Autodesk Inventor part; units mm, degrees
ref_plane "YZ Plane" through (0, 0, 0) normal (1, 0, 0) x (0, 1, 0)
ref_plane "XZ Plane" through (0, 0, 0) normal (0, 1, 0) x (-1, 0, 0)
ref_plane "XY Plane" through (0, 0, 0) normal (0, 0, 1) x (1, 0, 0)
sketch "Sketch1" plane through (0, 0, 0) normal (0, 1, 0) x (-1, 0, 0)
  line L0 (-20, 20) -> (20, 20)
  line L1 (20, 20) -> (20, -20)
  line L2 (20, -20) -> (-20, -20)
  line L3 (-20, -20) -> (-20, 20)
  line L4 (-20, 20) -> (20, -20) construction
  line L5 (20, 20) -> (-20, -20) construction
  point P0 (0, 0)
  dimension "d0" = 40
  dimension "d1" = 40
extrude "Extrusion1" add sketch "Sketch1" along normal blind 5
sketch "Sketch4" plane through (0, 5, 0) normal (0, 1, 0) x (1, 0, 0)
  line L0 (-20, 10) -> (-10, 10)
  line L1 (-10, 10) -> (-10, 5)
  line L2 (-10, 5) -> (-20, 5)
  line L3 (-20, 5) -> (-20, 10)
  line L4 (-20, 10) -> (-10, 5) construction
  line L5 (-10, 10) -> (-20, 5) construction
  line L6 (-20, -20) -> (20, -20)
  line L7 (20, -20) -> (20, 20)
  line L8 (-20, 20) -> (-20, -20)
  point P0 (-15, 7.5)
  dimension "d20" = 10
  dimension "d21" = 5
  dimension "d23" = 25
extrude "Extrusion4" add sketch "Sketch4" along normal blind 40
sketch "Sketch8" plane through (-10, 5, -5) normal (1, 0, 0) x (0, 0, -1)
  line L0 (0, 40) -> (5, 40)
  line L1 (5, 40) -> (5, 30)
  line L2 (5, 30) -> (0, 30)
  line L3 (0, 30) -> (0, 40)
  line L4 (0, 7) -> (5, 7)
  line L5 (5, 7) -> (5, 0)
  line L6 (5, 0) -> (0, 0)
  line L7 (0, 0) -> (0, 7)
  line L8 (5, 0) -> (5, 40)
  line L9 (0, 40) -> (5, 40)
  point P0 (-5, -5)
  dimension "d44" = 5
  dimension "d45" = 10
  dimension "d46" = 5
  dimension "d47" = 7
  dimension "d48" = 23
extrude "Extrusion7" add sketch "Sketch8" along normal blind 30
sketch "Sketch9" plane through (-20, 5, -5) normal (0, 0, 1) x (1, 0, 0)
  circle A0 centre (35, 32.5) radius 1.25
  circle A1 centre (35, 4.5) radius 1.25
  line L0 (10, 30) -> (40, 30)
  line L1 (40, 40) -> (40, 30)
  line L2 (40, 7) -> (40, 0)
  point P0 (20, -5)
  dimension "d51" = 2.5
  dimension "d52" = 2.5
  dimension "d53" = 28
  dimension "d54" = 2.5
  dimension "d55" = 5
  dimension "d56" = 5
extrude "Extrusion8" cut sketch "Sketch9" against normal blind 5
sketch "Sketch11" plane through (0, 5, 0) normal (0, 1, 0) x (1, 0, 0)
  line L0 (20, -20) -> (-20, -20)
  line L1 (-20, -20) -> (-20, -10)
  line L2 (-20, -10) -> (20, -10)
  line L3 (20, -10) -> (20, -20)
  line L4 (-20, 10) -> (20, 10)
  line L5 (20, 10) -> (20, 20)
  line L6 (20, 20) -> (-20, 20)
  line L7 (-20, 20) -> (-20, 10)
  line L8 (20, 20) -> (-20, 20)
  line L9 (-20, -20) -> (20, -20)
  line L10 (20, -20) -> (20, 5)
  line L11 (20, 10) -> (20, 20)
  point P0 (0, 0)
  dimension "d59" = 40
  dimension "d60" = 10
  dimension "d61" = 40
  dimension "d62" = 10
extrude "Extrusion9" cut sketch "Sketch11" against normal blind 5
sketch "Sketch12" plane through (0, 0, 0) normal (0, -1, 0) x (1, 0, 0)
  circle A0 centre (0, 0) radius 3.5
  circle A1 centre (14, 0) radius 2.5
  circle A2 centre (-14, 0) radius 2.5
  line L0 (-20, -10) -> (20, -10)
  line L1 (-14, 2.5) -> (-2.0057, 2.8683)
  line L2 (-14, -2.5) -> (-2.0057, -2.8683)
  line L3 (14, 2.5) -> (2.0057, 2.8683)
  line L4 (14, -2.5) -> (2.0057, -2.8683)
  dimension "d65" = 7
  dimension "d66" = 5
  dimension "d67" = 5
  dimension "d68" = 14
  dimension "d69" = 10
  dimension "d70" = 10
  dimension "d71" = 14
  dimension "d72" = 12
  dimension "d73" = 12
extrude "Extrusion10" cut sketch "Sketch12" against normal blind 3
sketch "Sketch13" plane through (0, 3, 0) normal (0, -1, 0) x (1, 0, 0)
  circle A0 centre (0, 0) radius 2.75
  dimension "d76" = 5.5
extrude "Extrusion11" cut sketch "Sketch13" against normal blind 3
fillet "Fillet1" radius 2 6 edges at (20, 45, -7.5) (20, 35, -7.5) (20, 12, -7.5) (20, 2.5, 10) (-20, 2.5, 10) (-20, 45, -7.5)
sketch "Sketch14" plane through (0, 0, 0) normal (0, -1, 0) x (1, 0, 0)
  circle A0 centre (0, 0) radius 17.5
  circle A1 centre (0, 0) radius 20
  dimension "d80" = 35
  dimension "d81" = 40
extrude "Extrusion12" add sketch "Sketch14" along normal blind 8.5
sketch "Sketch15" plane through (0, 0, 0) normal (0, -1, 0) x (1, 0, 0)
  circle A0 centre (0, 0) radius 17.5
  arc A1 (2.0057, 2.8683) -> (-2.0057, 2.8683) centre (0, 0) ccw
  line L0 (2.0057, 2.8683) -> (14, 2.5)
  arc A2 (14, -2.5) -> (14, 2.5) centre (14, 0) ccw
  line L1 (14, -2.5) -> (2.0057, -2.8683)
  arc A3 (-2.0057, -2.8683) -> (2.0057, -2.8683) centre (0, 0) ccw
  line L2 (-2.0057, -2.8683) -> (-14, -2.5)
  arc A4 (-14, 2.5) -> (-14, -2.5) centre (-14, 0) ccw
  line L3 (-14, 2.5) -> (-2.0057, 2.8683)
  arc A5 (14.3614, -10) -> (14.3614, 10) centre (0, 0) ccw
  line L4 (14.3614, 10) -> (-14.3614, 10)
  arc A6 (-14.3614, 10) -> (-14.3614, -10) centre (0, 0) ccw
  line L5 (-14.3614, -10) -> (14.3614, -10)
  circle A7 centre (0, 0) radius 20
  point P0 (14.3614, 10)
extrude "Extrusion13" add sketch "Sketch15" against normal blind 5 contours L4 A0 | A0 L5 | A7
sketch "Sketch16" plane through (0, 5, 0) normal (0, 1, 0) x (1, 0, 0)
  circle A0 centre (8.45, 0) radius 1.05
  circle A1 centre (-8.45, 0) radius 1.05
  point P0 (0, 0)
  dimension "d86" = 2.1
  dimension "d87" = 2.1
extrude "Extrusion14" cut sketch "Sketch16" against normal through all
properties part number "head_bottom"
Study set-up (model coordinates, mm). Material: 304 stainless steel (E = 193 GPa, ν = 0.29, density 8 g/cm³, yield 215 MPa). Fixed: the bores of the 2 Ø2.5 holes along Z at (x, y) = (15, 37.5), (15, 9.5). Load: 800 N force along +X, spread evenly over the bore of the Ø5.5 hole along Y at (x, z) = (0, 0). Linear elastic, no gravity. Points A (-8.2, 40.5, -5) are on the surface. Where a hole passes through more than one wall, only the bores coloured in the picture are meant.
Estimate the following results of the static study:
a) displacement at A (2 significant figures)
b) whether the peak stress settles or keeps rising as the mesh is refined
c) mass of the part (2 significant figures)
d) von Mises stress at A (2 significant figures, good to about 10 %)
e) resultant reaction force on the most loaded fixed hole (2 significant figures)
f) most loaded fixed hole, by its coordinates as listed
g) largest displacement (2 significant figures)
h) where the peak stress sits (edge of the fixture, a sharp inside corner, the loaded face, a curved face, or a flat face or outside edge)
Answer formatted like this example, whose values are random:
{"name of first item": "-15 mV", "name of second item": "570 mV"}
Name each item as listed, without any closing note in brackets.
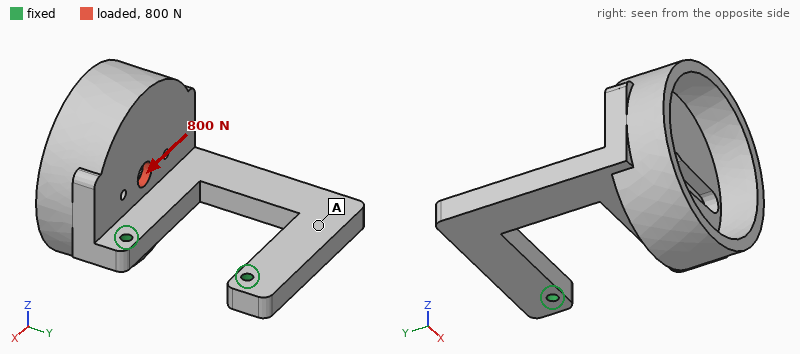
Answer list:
{"displacement at A": "9.7 µm", "whether the peak stress settles or keeps rising as the mesh is refined": "keeps rising", "mass of the part": "100 g", "von Mises stress at A": "10.0 MPa", "resultant reaction force on the most loaded fixed hole": "860 N", "most loaded fixed hole, by its coordinates as listed": "(15, 9.5)", "largest displacement": "44 µm", "where the peak stress sits": "edge of the fixture"}
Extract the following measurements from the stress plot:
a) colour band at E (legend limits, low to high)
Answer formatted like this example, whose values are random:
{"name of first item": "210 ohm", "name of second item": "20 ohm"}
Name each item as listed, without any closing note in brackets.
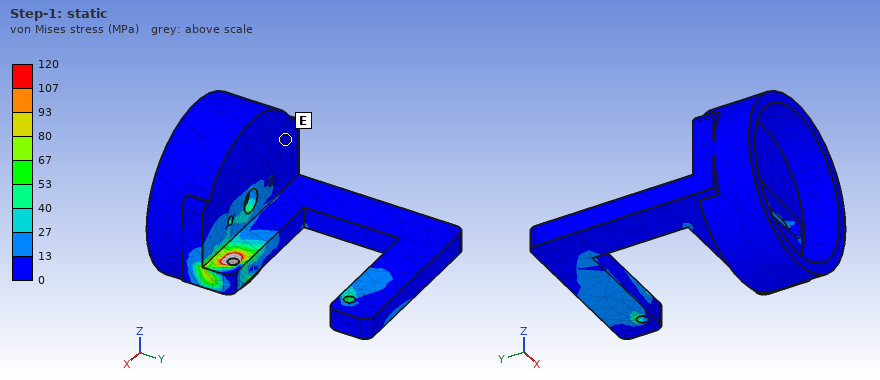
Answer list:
{"colour band at E": "0 to 13 MPa"}
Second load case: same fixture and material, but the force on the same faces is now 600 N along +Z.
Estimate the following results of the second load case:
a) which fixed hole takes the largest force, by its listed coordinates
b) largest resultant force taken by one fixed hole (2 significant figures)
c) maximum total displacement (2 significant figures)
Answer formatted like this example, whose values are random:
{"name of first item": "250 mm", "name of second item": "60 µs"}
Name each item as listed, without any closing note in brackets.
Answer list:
{"which fixed hole takes the largest force, by its listed coordinates": "(15, 9.5)", "largest resultant force taken by one fixed hole": "580 N", "maximum total displacement": "70 µm"}
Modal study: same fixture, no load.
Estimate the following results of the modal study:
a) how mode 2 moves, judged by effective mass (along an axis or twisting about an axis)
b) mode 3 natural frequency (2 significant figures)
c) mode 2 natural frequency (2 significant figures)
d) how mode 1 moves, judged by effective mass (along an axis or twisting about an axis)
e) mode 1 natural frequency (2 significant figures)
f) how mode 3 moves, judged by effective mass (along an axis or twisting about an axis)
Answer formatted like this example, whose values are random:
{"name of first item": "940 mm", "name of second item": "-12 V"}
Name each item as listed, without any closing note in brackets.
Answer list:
{"how mode 2 moves, judged by effective mass": "along Y", "mode 3 natural frequency": "3700 Hz", "mode 2 natural frequency": "2400 Hz", "how mode 1 moves, judged by effective mass": "along Z", "mode 1 natural frequency": "1700 Hz", "how mode 3 moves, judged by effective mass": "along Y"}
